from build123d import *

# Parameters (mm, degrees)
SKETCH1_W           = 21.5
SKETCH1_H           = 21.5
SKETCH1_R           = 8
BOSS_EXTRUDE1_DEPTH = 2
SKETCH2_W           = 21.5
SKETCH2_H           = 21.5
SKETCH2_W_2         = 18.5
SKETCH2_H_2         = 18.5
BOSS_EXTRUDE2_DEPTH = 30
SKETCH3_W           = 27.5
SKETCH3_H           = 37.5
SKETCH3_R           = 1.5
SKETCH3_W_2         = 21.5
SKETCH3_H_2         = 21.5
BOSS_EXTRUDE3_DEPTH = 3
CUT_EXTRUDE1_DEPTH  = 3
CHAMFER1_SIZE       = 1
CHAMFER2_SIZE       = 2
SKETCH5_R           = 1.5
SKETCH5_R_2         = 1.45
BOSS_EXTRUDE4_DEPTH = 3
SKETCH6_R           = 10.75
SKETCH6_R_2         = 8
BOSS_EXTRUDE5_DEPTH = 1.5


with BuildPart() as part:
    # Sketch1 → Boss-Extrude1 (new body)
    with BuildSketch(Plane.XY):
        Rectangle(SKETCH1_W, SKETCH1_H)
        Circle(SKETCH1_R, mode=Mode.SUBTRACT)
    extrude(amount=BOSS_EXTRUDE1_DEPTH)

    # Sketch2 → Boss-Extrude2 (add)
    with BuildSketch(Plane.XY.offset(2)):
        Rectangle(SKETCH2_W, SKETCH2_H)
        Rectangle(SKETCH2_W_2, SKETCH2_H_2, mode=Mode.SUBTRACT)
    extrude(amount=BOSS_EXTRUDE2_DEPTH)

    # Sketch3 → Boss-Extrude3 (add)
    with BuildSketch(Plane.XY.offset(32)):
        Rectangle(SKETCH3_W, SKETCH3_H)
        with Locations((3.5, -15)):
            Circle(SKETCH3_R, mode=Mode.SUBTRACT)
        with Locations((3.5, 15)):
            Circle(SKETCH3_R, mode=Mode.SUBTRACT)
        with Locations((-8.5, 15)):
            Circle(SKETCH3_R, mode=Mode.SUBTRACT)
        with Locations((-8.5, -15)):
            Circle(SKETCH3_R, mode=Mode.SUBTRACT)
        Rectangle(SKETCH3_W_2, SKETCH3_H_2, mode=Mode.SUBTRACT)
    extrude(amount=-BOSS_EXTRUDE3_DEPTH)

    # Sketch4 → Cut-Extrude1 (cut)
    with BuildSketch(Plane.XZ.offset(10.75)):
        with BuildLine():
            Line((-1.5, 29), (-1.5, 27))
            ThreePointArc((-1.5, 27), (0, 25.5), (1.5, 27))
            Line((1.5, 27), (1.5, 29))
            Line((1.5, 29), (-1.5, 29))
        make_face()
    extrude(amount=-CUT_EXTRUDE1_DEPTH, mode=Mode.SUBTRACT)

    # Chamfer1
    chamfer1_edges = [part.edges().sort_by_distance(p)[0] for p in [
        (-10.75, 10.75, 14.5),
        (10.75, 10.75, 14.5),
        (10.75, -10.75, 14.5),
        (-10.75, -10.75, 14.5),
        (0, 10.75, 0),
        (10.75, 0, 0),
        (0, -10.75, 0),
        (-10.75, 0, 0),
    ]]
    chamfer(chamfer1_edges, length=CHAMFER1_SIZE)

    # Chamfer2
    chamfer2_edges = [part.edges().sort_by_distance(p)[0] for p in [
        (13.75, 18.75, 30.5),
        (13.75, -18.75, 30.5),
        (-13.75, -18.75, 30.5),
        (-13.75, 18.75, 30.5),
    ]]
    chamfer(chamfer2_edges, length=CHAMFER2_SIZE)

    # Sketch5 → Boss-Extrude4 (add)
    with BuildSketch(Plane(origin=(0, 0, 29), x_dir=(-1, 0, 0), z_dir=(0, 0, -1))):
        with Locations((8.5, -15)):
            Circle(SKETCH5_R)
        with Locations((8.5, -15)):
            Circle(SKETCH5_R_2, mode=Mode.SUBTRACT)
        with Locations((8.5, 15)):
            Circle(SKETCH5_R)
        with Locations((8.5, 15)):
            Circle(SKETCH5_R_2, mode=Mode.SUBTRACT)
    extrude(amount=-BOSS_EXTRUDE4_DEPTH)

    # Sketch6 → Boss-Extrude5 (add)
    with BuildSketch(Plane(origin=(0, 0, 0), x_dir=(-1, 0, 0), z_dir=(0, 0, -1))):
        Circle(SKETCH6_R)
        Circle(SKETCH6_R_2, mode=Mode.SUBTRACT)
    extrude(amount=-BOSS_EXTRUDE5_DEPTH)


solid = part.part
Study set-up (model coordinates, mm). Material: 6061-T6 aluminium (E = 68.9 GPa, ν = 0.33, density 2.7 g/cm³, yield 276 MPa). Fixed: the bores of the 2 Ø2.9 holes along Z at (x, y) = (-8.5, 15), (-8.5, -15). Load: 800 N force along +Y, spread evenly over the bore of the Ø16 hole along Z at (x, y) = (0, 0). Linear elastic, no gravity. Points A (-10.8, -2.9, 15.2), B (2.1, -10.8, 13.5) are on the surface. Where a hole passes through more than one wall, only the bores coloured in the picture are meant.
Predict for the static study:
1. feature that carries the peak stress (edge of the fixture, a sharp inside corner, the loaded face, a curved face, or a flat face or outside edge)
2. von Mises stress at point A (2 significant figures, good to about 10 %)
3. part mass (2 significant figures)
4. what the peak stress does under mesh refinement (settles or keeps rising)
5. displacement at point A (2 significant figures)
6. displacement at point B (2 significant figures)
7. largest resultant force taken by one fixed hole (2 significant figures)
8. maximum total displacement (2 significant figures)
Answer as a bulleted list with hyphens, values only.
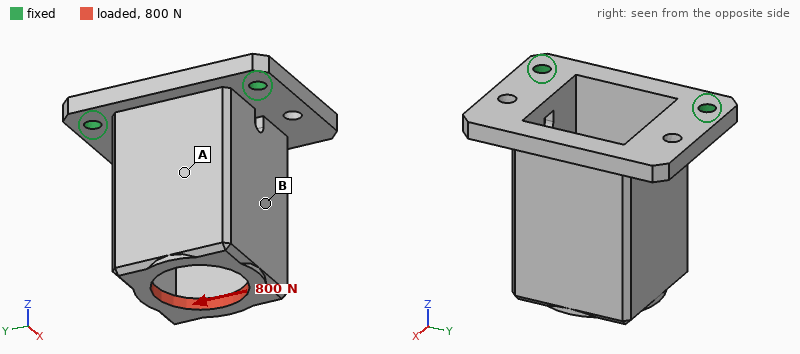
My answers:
- edge of the fixture
- 39 MPa
- 15 g
- keeps rising
- 0.041 mm
- 0.068 mm
- 1.1 kN
- 0.12 mm
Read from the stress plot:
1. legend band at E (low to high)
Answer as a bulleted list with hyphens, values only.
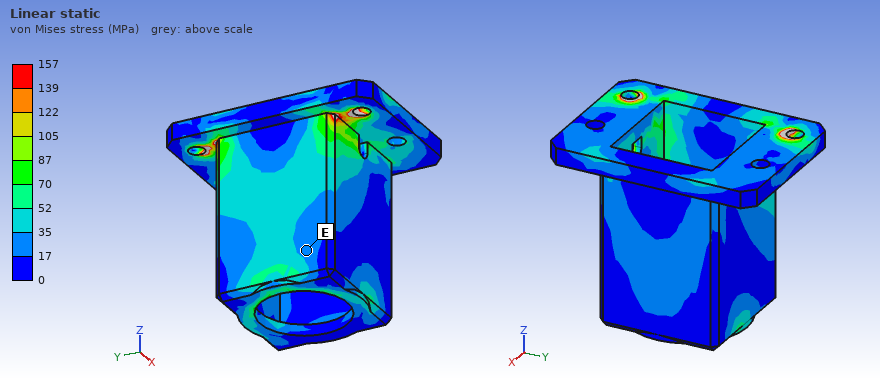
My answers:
- 17 to 35 MPa
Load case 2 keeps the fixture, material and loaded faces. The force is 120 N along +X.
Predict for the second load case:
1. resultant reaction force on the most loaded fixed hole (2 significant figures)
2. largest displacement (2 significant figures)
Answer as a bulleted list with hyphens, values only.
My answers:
- 61 N
- 0.13 mm
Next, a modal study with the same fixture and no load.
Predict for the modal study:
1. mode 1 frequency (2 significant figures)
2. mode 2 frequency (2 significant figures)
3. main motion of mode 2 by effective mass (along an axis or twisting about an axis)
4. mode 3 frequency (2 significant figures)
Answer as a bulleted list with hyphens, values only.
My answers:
- 2100 Hz
- 6100 Hz
- along Y
- 9000 Hz
